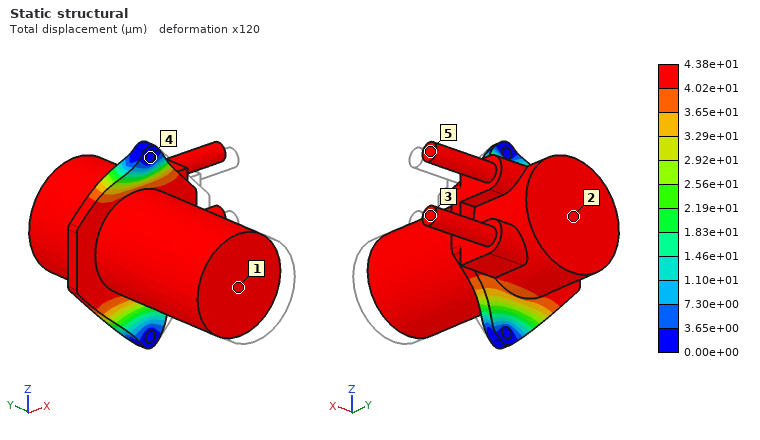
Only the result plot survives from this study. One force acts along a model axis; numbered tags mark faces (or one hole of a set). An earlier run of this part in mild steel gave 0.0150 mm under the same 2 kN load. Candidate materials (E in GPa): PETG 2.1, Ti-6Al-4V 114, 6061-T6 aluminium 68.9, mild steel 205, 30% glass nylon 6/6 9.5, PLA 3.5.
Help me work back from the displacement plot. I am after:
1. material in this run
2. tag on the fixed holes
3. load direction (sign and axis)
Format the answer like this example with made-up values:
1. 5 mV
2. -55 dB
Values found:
1. 6061-T6 aluminium
2. 4
3. +Y
